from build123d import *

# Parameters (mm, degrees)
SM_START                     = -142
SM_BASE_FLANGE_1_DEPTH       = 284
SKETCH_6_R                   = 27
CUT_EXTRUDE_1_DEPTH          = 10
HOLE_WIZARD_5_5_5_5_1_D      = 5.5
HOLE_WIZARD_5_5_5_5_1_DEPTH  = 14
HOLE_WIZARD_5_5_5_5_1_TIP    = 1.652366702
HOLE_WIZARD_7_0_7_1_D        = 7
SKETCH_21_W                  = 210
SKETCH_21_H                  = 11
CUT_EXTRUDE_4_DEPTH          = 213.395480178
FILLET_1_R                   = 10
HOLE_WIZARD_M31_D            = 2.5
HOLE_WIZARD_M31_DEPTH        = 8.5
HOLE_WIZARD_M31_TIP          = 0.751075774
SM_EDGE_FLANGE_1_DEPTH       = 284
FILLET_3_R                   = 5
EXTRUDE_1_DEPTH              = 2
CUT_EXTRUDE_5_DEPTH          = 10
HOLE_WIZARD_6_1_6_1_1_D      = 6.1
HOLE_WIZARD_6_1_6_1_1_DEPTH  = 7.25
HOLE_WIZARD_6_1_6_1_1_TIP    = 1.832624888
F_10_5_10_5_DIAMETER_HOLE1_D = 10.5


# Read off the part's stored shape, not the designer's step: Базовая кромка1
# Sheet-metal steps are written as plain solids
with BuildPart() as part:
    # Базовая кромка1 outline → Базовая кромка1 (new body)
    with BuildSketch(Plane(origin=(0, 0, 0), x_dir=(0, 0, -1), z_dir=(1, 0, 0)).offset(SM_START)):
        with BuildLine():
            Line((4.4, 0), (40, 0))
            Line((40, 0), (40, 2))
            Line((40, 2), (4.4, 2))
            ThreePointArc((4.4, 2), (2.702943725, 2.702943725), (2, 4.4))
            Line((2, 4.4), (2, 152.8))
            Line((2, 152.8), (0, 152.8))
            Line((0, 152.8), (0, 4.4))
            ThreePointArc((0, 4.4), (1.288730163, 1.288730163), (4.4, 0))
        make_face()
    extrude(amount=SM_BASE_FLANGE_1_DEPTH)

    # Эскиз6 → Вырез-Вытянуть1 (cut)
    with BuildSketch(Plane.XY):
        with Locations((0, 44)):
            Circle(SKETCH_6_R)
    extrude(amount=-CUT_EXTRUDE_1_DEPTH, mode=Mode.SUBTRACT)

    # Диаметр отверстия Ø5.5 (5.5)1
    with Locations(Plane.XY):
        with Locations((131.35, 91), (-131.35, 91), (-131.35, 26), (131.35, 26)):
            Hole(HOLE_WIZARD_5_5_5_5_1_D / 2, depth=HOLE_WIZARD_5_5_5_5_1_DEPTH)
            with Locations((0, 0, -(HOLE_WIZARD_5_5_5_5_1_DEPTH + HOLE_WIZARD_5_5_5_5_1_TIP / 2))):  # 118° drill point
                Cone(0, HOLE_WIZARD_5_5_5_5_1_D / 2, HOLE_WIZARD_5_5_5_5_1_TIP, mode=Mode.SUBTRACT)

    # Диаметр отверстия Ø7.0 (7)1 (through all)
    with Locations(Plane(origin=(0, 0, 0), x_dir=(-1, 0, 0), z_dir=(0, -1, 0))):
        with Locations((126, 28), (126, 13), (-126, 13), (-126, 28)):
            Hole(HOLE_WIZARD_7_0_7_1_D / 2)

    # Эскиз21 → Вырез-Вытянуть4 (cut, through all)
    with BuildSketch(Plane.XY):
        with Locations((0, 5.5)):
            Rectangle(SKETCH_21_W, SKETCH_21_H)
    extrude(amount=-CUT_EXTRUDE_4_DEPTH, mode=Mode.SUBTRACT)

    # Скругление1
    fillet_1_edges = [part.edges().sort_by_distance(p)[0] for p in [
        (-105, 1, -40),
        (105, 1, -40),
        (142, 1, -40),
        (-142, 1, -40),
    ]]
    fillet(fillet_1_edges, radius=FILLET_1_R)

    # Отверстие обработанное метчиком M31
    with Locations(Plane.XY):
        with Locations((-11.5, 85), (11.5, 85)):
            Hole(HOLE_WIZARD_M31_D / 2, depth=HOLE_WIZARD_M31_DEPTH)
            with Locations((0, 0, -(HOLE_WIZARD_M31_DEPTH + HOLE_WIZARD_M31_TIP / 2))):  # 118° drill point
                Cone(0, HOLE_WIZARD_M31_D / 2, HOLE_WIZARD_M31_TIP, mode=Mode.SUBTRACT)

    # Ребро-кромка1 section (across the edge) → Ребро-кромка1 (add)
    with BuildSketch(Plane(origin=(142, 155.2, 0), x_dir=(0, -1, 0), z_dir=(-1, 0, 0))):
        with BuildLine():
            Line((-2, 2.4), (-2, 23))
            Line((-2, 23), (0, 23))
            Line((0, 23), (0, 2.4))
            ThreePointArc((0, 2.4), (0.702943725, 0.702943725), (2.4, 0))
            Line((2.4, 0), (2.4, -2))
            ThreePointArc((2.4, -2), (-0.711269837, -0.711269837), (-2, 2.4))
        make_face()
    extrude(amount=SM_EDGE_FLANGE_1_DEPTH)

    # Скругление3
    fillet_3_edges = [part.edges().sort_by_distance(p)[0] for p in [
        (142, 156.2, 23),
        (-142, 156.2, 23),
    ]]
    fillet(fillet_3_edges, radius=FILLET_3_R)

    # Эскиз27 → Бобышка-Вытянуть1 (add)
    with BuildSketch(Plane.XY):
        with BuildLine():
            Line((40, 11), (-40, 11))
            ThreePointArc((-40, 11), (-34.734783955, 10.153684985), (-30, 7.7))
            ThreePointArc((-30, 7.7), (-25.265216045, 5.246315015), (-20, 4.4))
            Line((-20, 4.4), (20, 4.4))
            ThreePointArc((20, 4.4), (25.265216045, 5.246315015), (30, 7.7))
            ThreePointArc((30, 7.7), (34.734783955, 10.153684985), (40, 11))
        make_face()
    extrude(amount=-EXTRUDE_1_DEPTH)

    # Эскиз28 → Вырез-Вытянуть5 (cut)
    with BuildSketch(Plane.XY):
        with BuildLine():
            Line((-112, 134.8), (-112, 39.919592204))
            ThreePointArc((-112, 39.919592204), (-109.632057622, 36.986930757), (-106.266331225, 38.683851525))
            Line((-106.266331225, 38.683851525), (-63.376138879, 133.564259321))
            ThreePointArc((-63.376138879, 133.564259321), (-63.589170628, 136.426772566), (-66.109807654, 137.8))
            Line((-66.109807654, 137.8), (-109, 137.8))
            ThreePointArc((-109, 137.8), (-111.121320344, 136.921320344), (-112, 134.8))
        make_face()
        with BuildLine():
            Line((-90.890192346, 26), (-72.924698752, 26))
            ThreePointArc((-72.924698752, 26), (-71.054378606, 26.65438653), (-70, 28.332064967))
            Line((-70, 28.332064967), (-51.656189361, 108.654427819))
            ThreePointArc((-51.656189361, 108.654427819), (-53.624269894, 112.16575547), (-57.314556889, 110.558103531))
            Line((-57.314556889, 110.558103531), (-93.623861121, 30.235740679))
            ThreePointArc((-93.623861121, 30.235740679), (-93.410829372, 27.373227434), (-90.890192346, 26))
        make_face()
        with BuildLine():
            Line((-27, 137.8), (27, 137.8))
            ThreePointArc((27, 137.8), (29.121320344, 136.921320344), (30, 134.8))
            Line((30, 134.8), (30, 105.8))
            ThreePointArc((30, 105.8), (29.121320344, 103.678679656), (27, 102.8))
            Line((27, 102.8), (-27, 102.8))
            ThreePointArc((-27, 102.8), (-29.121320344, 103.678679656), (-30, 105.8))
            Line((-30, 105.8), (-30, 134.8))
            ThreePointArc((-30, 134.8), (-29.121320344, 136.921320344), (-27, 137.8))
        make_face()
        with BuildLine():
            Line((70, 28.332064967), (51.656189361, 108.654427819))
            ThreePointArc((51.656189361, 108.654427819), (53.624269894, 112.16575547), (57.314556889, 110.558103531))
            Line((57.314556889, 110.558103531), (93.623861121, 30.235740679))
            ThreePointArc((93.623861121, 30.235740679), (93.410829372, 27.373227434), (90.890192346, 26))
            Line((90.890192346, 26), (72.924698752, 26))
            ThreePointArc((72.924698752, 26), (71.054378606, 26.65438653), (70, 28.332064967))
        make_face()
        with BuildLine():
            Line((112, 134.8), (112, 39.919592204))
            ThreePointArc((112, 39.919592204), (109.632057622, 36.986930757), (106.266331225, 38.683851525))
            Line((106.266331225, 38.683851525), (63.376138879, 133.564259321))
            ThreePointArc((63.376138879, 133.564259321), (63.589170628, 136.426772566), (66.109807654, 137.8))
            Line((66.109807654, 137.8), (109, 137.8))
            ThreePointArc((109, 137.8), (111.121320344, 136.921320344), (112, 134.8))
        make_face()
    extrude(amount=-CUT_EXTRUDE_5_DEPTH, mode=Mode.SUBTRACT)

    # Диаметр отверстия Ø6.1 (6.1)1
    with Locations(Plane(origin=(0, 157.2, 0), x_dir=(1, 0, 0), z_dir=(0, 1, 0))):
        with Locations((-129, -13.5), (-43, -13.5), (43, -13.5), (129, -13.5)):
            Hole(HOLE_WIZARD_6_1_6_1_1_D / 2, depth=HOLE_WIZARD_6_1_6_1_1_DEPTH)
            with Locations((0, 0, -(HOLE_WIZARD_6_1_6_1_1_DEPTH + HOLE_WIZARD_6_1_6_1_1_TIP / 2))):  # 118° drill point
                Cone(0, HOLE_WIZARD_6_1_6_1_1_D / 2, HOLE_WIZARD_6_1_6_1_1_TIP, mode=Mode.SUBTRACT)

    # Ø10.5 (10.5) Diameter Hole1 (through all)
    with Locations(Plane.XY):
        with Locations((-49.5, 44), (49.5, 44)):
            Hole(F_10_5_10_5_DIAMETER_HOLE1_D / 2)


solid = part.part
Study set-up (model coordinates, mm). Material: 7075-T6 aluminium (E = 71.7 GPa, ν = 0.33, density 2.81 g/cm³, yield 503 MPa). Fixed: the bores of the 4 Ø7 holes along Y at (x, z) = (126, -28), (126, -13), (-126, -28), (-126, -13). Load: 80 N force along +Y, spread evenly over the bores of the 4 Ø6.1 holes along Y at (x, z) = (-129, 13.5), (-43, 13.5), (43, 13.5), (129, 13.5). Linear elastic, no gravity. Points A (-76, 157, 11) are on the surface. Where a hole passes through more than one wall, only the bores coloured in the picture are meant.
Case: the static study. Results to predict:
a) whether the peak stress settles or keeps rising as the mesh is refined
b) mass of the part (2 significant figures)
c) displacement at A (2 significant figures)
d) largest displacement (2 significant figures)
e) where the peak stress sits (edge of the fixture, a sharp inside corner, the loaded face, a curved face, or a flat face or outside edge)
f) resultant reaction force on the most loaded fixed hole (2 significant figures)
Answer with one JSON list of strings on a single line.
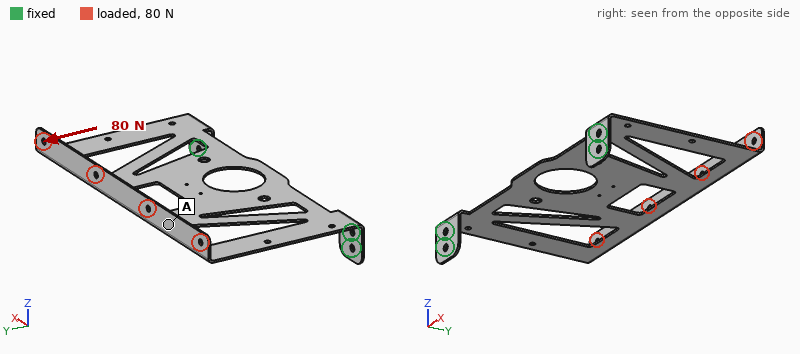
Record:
["keeps rising", "220 g", "3.3 mm", "3.4 mm", "edge of the fixture", "57 N"]
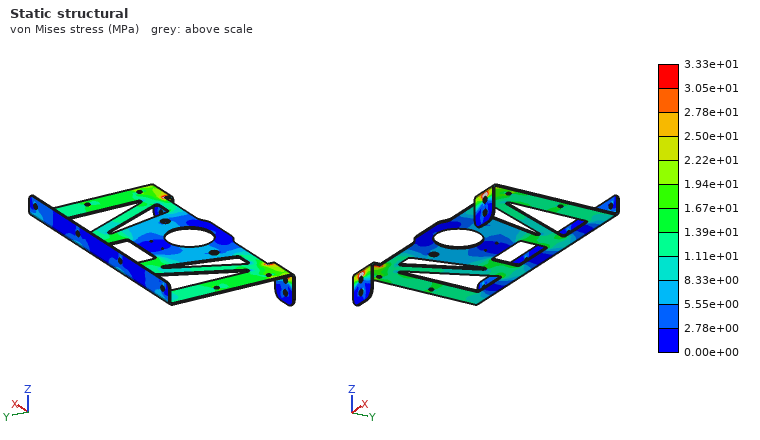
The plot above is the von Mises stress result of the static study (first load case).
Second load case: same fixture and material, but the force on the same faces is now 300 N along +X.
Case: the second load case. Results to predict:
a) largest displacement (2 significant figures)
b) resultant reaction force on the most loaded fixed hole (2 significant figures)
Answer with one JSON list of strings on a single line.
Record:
["3.8 mm", "290 N"]
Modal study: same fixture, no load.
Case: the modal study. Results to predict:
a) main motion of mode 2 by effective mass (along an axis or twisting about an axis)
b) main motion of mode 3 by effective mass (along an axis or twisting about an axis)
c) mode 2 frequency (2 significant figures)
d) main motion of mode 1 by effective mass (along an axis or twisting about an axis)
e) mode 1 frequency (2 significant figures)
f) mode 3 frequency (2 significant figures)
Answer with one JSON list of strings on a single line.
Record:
["twisting about Y", "along Z", "79 Hz", "along Z", "31 Hz", "170 Hz"]
